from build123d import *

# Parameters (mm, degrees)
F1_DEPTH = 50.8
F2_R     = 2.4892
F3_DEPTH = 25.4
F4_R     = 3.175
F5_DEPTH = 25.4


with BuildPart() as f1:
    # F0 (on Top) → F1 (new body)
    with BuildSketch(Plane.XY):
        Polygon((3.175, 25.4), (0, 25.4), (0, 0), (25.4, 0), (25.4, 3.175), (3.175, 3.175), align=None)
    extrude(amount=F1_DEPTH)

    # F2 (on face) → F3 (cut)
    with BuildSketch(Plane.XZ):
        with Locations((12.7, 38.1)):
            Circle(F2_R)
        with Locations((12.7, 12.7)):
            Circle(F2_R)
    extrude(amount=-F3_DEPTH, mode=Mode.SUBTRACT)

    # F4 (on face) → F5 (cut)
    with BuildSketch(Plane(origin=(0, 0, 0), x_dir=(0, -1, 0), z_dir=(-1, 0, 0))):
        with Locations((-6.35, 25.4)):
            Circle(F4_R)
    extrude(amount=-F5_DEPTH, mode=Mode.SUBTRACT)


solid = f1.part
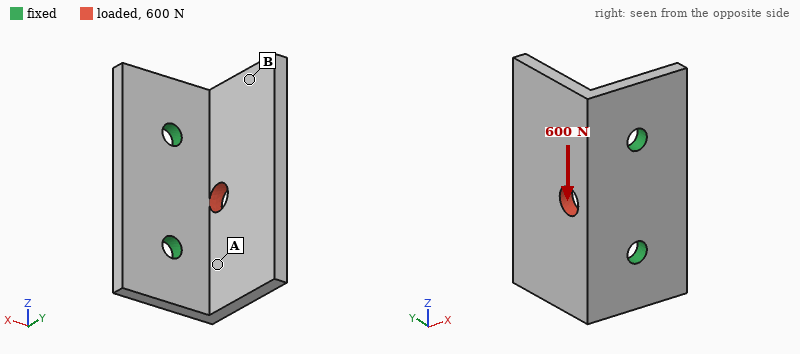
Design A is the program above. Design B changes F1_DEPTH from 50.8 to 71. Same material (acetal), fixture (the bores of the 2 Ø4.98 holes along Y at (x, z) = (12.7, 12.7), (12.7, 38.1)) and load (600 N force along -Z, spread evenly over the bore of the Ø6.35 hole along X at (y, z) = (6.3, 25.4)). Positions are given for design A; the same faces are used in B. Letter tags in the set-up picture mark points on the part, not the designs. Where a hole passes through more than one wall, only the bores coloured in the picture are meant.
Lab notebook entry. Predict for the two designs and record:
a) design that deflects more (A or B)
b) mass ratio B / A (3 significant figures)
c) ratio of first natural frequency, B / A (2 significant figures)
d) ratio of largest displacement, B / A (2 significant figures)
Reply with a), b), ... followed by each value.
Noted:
a) B
b) 1.41
c) 0.87
d) 1.3
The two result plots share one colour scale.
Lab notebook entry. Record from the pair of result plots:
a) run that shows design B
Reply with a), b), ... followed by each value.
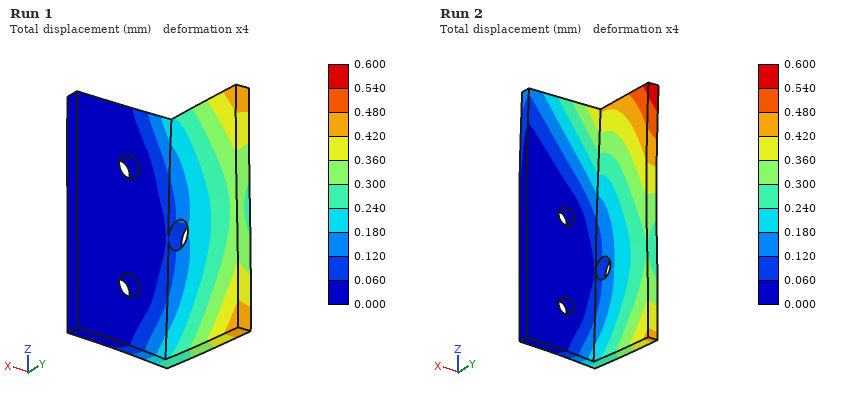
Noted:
a) Run 2
